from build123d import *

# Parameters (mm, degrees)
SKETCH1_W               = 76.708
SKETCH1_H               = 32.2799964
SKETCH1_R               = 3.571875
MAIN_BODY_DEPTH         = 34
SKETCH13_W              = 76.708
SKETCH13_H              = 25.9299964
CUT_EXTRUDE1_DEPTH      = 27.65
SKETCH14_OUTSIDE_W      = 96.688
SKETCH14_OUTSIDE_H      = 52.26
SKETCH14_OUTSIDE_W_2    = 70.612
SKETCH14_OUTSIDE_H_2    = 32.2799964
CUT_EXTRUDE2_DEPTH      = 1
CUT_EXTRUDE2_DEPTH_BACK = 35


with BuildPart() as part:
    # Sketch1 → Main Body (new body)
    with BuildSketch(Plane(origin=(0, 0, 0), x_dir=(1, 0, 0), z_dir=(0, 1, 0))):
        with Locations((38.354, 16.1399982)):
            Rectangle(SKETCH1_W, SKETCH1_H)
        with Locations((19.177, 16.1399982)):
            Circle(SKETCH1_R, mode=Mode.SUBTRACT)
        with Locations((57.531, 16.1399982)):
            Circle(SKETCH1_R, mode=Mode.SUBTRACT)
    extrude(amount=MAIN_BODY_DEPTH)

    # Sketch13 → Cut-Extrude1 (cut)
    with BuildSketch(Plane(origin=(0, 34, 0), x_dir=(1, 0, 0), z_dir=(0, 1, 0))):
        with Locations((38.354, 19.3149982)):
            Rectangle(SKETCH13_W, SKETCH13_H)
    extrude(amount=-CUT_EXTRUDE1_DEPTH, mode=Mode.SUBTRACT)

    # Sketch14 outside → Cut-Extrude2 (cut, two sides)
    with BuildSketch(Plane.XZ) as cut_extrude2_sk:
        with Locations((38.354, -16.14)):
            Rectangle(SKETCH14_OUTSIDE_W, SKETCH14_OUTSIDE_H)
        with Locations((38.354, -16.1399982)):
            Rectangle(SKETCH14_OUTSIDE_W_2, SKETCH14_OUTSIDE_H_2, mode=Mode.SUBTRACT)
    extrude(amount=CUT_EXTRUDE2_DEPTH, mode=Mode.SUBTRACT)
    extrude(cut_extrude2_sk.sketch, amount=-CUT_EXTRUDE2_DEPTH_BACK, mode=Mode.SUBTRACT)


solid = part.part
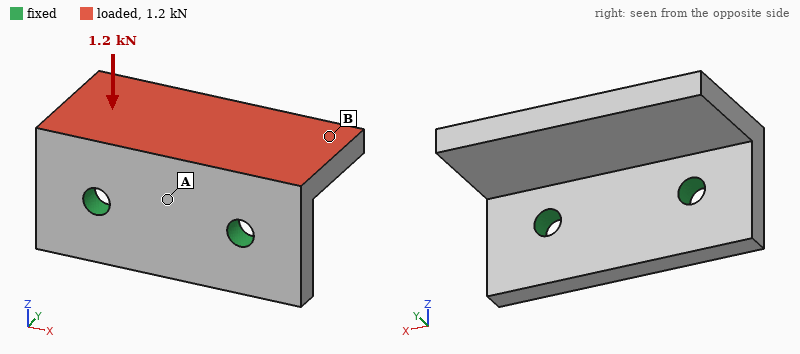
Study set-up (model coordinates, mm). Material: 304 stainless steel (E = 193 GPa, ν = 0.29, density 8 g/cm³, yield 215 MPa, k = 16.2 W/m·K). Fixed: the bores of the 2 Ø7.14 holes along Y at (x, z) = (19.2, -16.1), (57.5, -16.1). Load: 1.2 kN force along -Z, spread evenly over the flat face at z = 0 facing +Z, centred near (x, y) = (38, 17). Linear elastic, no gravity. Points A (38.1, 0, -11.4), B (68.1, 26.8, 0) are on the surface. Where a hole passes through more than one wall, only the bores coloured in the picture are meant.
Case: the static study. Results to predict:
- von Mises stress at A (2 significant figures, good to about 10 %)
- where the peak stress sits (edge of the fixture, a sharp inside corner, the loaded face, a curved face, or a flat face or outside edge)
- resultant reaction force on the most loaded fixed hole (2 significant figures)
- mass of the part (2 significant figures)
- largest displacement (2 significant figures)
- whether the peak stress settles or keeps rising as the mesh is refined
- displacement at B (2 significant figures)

20 MPa
edge of the fixture
600 N
210 g
33 µm
keeps rising
25 µm
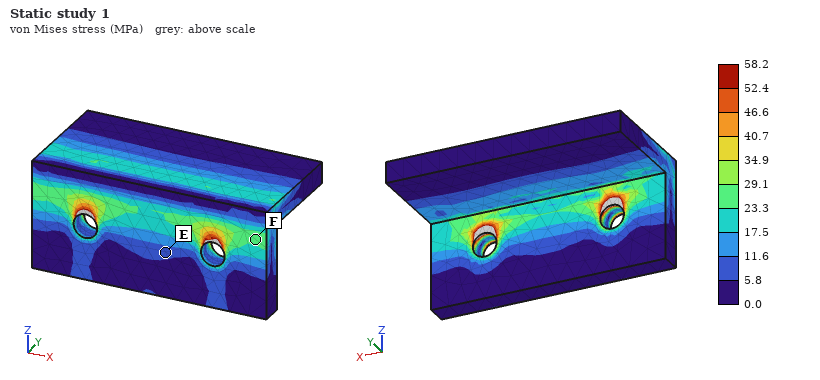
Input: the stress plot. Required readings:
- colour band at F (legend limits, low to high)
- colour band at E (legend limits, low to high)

23.3 to 29.1 MPa
5.8 to 11.6 MPa
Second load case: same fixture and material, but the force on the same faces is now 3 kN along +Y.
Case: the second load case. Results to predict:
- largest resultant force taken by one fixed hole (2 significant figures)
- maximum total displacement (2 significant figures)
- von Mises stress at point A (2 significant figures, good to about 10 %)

1.5 kN
50 µm
33 MPa
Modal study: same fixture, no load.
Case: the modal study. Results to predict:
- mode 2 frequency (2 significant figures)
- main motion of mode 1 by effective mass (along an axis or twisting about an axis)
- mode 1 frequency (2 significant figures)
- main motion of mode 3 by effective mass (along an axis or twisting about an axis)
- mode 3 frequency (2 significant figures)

5300 Hz
along Z
3300 Hz
along X
8900 Hz
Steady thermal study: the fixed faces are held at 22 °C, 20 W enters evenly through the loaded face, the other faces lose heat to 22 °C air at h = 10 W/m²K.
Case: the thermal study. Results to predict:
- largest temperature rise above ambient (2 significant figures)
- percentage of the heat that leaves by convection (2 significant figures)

66 K
11 %
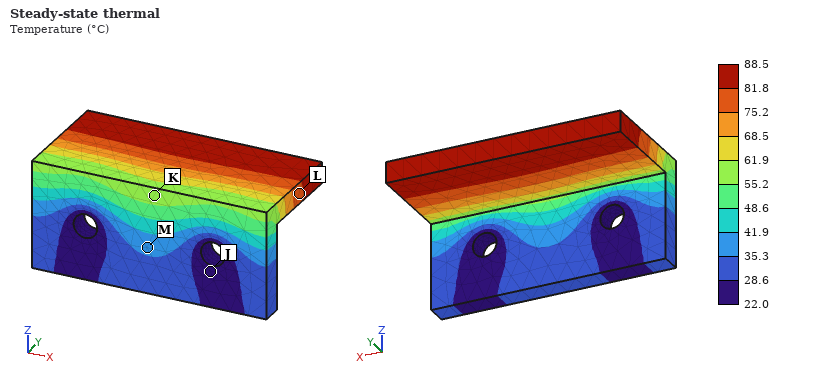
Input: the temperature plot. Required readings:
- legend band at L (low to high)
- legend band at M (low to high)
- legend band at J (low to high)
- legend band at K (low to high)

75.2 to 81.8 °C
35.3 to 41.9 °C
22.0 to 28.6 °C
55.2 to 61.9 °C
